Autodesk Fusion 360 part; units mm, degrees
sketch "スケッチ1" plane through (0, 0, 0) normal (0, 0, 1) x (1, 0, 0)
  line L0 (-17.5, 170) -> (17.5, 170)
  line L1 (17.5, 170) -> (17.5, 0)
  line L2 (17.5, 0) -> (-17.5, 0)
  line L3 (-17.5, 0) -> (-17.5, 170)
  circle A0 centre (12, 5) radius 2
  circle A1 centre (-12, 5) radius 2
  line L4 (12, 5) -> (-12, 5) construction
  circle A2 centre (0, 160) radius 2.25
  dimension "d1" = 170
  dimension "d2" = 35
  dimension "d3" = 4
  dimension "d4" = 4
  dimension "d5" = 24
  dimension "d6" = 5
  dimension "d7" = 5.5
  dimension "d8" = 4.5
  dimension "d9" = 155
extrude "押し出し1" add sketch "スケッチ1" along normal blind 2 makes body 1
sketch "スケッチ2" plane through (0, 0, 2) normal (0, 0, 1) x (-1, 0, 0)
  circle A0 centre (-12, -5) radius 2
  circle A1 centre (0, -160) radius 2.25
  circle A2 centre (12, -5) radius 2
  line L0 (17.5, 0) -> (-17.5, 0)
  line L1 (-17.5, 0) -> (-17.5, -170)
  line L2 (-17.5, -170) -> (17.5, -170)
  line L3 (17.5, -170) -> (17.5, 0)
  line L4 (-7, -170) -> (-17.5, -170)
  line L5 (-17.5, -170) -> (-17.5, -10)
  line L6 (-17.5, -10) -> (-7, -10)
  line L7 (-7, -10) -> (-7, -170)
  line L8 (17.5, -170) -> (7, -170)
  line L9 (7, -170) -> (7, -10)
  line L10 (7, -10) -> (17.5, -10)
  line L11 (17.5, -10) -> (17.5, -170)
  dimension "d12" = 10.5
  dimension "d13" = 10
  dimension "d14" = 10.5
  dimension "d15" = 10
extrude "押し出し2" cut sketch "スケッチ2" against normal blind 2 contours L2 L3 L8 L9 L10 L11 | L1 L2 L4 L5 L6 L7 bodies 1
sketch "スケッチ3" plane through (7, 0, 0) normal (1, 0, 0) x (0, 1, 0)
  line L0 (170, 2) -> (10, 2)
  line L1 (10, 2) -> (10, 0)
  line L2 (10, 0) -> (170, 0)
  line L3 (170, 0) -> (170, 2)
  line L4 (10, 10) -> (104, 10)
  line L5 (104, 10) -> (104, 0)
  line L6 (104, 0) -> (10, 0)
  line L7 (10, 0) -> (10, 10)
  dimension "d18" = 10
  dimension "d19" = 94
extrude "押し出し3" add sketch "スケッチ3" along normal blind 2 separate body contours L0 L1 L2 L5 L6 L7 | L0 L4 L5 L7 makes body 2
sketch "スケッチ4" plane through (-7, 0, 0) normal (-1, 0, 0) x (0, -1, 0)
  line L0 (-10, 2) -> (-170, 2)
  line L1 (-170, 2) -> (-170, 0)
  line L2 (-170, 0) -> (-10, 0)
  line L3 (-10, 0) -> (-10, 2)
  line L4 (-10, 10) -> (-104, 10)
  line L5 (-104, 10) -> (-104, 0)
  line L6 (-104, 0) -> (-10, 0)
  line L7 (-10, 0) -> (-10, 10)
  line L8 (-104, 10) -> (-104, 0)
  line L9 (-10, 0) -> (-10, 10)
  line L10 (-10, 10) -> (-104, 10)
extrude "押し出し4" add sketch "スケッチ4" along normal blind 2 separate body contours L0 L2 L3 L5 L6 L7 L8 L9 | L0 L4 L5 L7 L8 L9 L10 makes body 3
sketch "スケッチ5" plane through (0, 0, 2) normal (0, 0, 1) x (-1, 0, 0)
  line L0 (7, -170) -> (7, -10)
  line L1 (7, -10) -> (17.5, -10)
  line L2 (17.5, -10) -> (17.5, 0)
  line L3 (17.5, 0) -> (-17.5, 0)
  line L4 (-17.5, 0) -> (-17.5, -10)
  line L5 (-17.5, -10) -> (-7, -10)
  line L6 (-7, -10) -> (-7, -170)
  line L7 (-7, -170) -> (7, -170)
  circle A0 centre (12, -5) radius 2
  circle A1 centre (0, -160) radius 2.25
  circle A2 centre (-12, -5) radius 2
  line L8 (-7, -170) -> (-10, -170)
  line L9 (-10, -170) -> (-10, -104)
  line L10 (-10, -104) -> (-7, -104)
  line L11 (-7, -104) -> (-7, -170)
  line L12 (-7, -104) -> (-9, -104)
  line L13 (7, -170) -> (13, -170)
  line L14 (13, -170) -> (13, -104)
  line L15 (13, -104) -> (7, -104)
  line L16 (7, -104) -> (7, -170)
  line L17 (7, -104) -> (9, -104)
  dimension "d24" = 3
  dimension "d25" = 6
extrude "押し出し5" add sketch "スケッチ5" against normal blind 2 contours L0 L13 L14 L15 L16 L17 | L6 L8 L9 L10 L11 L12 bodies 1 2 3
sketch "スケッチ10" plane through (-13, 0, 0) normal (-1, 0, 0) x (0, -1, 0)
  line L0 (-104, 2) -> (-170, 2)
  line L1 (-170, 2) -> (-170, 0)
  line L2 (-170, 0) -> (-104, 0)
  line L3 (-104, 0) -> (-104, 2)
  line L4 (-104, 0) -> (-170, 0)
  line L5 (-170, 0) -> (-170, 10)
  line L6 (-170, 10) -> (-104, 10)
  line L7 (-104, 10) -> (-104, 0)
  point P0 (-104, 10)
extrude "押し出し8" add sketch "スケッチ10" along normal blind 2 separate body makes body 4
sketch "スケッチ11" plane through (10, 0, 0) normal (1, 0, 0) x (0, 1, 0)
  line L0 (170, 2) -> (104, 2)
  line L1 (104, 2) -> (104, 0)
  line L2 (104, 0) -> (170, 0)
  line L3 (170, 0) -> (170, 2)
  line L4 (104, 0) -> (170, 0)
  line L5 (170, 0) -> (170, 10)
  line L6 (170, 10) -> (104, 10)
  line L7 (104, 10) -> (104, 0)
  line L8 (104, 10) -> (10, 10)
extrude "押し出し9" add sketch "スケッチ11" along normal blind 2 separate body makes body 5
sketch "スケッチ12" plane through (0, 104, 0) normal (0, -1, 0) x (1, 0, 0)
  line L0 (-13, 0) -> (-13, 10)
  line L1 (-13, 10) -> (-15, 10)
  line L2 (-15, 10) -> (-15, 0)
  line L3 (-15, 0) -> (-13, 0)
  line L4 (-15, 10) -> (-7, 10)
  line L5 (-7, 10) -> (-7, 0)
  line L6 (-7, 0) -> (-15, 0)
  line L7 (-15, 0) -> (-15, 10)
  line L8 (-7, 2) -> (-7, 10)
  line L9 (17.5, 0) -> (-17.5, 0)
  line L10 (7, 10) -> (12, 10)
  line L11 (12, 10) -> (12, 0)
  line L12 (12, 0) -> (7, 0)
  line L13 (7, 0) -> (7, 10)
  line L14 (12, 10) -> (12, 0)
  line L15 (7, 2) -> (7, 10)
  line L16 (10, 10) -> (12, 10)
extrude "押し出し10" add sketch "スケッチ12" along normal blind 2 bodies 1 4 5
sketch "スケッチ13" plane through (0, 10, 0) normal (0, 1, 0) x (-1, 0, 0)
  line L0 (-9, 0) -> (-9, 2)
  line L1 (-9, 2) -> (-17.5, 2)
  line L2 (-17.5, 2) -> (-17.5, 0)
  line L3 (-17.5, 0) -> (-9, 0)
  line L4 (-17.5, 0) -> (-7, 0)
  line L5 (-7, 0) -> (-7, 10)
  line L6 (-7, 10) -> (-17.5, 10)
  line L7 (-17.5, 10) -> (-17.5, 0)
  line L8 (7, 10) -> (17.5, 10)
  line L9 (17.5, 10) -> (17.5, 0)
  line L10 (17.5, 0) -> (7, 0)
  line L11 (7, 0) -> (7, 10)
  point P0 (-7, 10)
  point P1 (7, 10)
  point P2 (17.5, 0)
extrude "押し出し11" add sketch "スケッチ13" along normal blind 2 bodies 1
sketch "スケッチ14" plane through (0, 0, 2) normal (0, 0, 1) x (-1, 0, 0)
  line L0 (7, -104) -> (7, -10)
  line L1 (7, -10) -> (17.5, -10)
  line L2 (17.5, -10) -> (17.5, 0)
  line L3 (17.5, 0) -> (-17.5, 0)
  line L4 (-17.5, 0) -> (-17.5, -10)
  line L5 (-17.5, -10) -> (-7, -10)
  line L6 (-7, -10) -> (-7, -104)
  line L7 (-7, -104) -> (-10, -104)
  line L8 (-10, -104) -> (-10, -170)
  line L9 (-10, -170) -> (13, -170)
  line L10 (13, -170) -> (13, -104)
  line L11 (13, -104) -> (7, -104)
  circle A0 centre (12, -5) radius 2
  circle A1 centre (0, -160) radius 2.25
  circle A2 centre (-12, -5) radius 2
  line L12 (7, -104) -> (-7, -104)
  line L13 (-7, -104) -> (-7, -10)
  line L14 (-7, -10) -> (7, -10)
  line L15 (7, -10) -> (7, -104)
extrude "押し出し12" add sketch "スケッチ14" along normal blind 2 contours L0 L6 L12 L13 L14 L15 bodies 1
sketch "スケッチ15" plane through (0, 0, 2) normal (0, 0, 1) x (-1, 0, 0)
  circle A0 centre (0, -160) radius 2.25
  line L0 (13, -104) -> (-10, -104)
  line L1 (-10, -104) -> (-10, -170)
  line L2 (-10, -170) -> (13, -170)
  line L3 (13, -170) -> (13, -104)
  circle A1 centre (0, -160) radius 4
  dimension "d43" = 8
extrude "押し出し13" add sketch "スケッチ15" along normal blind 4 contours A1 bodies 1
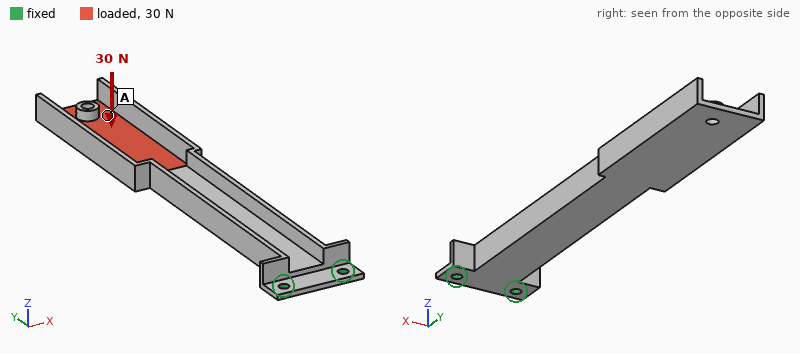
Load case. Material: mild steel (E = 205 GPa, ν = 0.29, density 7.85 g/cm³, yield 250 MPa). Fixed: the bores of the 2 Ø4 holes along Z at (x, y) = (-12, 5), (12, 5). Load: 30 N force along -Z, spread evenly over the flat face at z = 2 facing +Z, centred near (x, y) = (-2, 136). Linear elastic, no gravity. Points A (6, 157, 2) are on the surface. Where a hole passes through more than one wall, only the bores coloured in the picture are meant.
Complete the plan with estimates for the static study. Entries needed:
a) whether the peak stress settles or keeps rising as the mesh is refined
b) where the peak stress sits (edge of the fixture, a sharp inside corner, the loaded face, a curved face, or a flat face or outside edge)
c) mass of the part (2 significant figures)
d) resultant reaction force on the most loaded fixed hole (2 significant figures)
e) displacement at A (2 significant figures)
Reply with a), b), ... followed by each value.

a) keeps rising
b) edge of the fixture
c) 130 g
d) 73 N
e) 0.99 mm
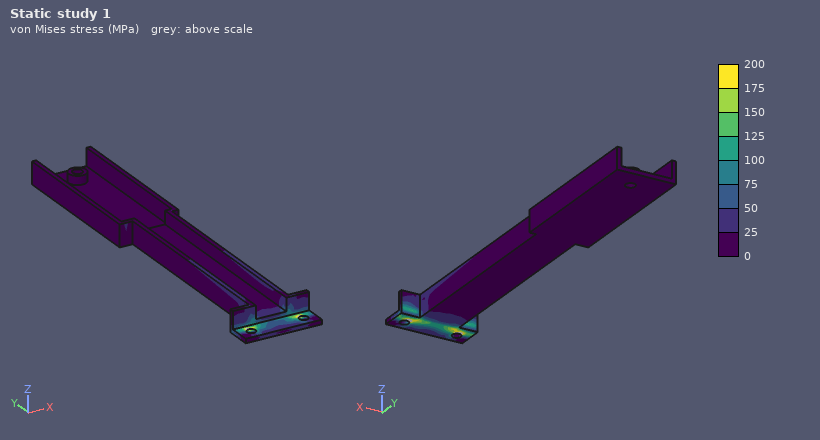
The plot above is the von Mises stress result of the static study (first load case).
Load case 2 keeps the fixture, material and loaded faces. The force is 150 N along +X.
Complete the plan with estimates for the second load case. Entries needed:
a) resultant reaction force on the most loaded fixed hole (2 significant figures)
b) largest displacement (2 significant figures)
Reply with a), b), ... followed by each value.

a) 870 N
b) 0.32 mm
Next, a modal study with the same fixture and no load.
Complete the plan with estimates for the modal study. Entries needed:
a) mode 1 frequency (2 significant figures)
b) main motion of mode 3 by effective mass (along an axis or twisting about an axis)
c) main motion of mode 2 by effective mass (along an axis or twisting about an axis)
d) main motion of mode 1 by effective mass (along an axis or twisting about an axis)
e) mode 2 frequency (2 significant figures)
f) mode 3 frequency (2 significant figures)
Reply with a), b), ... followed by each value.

a) 120 Hz
b) twisting about Y
c) along X
d) along Z
e) 530 Hz
f) 1000 Hz
